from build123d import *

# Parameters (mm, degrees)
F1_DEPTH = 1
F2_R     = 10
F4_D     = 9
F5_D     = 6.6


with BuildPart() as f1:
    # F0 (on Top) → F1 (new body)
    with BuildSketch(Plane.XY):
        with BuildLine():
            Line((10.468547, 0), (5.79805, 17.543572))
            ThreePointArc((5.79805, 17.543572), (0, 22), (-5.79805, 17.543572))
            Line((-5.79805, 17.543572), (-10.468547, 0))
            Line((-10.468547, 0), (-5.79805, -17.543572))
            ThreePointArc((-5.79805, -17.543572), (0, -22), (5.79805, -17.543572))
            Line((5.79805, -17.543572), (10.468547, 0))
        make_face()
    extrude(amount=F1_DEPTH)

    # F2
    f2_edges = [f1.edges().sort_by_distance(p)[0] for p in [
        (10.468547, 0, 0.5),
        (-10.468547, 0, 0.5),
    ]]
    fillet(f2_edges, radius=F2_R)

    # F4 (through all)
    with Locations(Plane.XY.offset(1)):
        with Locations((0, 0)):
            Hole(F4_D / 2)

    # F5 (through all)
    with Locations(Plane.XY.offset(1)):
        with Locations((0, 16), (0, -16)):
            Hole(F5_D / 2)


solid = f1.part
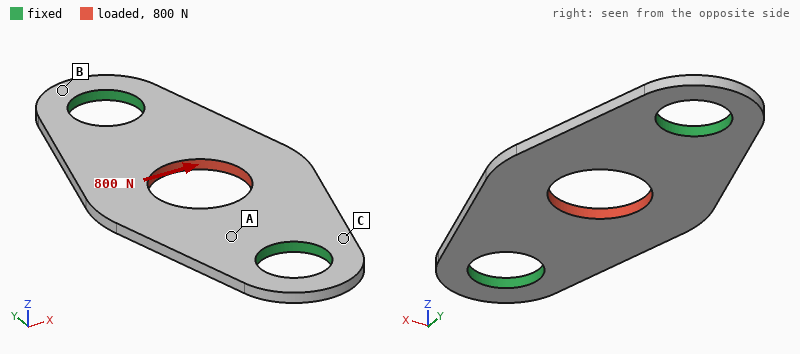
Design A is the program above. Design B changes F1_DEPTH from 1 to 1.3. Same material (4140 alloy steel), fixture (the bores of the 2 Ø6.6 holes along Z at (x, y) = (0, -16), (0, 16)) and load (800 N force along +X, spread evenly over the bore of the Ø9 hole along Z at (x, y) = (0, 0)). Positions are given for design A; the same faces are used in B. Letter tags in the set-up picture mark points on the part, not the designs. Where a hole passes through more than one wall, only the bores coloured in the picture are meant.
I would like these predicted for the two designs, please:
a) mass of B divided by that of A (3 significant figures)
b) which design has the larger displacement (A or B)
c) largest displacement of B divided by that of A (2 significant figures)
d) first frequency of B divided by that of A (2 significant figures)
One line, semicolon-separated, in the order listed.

1.30; A; 0.77; 1.3
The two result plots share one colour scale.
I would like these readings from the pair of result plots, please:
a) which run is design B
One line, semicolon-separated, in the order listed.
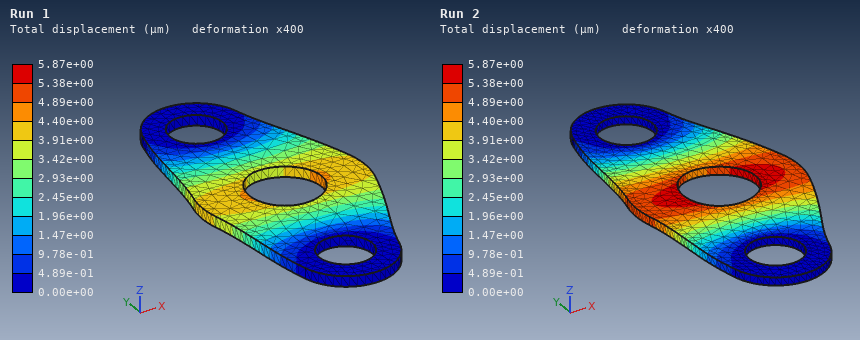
Run 1
